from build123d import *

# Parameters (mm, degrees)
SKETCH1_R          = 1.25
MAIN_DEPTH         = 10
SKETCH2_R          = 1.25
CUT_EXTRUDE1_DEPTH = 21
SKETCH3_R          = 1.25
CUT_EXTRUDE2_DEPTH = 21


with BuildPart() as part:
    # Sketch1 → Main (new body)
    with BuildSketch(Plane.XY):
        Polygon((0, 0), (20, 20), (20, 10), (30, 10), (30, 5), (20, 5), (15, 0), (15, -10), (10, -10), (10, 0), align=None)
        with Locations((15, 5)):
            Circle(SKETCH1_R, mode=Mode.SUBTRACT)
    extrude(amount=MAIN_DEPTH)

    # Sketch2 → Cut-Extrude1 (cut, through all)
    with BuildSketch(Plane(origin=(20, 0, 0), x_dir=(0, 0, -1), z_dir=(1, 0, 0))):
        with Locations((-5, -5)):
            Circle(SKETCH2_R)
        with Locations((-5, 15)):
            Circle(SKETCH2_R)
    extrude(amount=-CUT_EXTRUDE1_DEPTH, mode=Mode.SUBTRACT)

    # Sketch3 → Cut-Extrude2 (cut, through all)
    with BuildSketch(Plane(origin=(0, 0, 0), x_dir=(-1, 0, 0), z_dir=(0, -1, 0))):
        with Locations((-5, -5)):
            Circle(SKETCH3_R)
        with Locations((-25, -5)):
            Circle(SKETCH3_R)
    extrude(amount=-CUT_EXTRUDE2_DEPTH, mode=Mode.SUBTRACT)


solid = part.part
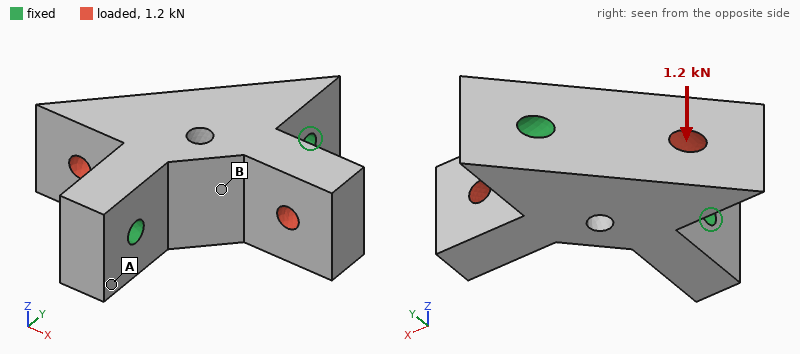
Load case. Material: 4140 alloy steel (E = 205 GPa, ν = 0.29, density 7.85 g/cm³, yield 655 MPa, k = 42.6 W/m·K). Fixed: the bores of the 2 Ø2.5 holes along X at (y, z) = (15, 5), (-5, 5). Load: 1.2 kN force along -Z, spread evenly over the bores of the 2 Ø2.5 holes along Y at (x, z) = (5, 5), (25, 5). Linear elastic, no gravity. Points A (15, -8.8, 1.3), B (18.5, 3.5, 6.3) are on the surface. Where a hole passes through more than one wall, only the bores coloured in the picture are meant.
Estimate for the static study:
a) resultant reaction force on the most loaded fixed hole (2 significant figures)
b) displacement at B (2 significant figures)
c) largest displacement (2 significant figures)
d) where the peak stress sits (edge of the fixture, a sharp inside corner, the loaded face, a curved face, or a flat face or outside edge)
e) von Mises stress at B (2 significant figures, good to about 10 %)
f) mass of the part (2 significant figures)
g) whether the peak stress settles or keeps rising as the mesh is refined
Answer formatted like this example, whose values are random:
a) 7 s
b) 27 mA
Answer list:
a) 620 N
b) 2.6 µm
c) 8.3 µm
d) edge of the fixture
e) 38 MPa
f) 21 g
g) keeps rising
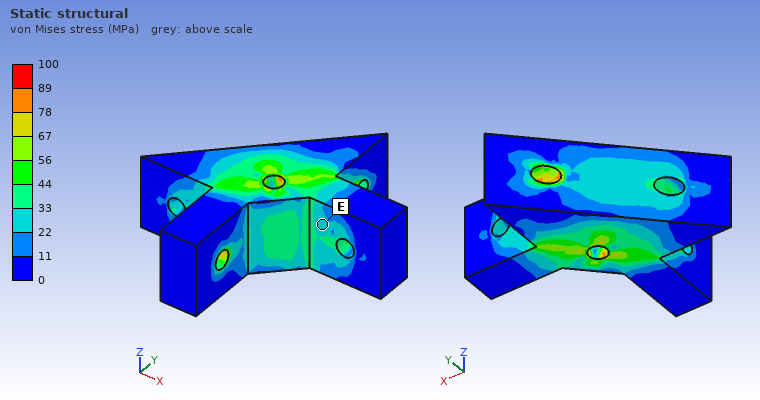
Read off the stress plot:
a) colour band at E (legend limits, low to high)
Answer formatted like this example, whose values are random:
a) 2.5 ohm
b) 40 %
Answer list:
a) 22 to 33 MPa
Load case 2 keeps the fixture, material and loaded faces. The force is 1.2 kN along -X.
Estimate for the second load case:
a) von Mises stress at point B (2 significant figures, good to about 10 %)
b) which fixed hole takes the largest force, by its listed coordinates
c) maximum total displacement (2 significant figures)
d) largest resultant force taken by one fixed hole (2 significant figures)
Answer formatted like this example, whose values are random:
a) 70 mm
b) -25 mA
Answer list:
a) 16 MPa
b) (15, 5)
c) 2.7 µm
d) 670 N
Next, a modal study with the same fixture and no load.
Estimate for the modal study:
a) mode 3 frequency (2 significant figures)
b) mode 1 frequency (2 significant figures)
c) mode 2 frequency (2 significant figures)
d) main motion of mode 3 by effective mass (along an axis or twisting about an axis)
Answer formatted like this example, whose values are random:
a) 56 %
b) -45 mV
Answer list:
a) 28 kHz
b) 18 kHz
c) 24 kHz
d) along Z
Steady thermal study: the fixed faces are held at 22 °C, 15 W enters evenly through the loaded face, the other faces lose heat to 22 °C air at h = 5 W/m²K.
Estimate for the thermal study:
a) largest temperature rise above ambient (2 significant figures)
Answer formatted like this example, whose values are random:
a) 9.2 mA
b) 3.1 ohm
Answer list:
a) 49 K
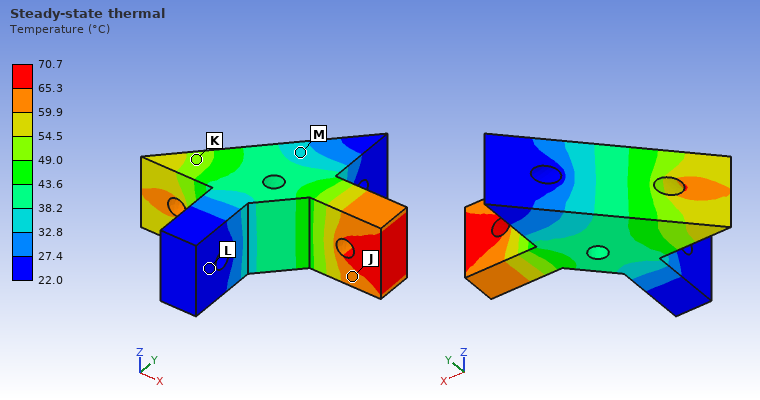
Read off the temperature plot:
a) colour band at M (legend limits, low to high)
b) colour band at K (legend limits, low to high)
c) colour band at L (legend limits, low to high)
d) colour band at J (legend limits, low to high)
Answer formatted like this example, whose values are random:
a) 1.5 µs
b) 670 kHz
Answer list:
a) 32.8 to 38.2 °C
b) 49.0 to 54.5 °C
c) 22.0 to 27.4 °C
d) 59.9 to 65.3 °C
